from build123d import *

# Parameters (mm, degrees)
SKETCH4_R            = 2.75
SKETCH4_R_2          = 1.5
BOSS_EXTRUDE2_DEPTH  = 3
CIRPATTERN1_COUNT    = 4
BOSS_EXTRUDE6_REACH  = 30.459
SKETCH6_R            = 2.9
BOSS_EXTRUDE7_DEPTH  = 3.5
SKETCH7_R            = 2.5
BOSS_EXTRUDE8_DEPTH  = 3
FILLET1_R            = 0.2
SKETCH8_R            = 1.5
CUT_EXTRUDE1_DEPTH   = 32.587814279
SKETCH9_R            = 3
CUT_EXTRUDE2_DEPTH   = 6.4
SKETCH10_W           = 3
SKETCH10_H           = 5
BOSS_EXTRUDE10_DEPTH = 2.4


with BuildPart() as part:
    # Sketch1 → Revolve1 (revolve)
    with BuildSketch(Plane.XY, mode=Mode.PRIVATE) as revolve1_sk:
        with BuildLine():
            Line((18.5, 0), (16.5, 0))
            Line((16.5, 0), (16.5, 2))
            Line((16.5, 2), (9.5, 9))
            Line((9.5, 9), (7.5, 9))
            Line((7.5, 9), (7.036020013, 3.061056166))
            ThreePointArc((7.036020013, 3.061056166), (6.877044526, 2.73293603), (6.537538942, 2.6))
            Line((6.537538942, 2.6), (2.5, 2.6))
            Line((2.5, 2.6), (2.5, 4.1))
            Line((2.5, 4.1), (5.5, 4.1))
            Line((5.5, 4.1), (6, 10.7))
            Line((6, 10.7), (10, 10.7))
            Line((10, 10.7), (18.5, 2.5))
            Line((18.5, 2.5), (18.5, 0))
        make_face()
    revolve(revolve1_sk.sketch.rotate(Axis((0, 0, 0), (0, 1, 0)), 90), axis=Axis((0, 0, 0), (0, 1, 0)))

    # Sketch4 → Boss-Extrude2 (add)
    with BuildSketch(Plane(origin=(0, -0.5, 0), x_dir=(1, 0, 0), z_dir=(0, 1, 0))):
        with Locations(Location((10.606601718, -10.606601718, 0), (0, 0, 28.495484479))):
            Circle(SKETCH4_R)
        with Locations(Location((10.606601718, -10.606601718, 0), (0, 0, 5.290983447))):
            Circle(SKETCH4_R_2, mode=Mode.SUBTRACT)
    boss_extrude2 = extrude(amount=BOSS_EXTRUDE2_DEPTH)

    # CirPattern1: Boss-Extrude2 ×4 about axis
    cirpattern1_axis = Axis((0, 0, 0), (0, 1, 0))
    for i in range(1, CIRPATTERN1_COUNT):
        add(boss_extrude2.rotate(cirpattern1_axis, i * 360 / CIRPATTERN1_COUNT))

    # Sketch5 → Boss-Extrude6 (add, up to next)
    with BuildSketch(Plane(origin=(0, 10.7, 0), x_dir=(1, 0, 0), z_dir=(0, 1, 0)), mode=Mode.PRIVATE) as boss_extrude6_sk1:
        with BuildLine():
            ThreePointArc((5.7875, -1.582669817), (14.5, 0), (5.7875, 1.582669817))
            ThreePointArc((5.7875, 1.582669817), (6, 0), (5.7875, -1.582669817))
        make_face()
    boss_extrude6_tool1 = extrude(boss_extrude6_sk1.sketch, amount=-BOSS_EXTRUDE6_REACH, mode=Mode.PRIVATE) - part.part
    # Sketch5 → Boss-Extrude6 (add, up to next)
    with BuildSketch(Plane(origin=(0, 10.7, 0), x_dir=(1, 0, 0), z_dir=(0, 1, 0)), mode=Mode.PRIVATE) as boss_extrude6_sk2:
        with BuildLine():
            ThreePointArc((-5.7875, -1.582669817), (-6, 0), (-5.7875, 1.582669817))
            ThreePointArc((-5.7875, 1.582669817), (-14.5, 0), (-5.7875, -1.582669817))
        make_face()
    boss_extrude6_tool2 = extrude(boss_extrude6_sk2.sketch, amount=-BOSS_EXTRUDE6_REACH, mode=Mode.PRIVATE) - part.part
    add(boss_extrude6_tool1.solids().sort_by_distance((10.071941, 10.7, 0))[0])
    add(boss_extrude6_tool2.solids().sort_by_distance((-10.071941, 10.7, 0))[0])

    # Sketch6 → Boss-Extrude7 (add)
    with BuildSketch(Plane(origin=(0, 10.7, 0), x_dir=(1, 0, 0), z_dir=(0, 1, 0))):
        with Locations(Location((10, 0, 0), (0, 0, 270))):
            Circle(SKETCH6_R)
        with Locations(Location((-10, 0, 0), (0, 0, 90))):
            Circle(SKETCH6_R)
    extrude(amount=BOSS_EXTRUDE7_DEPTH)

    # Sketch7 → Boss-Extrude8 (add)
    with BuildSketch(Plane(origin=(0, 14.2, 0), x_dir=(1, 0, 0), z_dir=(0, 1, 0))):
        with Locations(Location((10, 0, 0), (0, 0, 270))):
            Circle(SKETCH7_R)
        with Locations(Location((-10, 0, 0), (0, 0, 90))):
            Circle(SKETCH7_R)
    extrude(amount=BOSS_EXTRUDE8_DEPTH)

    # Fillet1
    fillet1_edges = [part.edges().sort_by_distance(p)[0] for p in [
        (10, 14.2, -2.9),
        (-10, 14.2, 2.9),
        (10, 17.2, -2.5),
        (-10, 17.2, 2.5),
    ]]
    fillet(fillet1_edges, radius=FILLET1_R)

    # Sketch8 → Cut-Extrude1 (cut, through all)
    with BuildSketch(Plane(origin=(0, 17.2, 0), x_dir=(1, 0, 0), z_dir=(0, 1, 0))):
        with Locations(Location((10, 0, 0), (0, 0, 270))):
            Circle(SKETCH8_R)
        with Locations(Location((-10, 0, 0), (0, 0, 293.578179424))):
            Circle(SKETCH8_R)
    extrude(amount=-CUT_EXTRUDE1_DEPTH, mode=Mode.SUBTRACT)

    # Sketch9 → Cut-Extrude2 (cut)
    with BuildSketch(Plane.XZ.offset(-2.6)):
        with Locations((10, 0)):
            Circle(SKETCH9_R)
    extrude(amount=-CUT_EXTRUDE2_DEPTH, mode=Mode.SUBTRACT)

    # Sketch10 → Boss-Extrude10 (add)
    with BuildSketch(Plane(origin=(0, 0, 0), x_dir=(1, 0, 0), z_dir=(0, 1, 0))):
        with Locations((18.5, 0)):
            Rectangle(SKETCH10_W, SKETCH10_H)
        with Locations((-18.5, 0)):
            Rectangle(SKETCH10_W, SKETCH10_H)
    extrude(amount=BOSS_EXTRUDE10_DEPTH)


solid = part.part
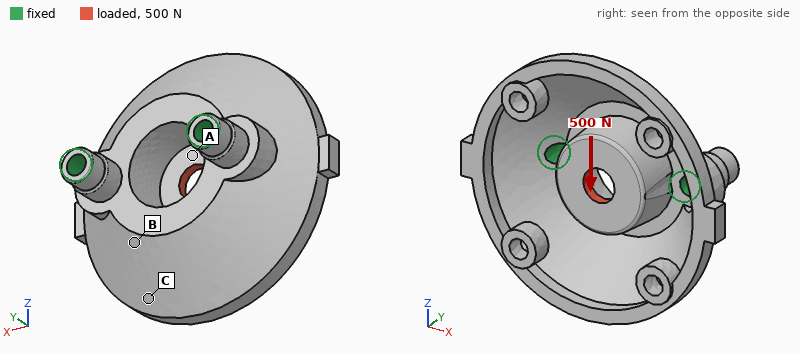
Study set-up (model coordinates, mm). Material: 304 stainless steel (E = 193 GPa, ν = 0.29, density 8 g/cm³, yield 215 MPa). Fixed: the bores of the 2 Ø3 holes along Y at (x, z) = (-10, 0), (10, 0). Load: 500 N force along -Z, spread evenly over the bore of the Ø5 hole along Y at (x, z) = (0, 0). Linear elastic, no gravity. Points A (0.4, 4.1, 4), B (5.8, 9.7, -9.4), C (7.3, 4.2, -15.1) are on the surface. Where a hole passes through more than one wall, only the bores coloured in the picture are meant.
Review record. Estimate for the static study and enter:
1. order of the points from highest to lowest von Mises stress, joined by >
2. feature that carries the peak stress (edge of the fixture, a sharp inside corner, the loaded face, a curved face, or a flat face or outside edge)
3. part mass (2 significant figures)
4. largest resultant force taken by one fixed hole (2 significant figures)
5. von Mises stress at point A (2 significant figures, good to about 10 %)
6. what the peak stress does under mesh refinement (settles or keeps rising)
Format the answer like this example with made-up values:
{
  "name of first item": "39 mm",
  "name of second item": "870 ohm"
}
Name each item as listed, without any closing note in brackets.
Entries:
{
  "order of the points from highest to lowest von Mises stress, joined by >": "A > B > C",
  "feature that carries the peak stress": "edge of the fixture",
  "part mass": "27 g",
  "largest resultant force taken by one fixed hole": "260 N",
  "von Mises stress at point A": "26 MPa",
  "what the peak stress does under mesh refinement": "keeps rising"
}
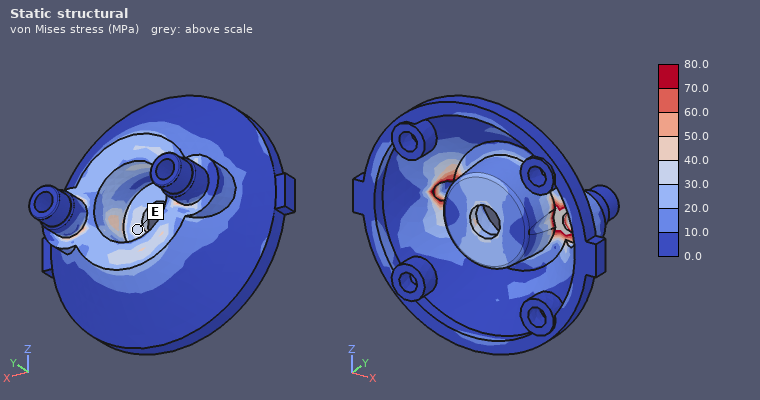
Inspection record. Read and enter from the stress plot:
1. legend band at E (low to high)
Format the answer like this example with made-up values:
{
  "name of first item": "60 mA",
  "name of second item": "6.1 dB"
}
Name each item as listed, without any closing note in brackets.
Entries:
{
  "legend band at E": "30.0 to 40.0 MPa"
}
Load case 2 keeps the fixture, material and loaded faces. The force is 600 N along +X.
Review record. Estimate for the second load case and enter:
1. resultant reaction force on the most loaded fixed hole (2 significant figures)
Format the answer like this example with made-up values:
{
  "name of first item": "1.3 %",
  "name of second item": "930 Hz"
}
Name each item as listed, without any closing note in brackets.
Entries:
{
  "resultant reaction force on the most loaded fixed hole": "390 N"
}
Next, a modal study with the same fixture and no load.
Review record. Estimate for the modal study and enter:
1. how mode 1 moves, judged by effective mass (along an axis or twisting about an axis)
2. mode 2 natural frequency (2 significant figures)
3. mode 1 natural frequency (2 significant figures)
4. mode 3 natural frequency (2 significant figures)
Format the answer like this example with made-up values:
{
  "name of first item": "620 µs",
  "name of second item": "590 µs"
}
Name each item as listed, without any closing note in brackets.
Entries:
{
  "how mode 1 moves, judged by effective mass": "along Z",
  "mode 2 natural frequency": "9000 Hz",
  "mode 1 natural frequency": "6800 Hz",
  "mode 3 natural frequency": "9200 Hz"
}
